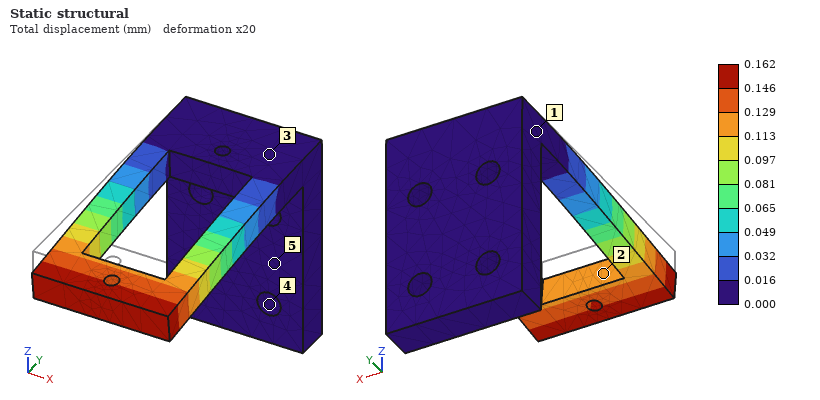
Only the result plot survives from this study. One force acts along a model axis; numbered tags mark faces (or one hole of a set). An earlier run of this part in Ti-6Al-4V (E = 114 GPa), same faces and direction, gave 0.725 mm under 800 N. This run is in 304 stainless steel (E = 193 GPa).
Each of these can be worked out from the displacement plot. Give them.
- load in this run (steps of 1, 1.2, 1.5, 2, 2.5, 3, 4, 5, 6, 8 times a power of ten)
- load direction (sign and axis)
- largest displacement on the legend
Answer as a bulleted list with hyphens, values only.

- 300 N
- -Z
- 0.162 mm
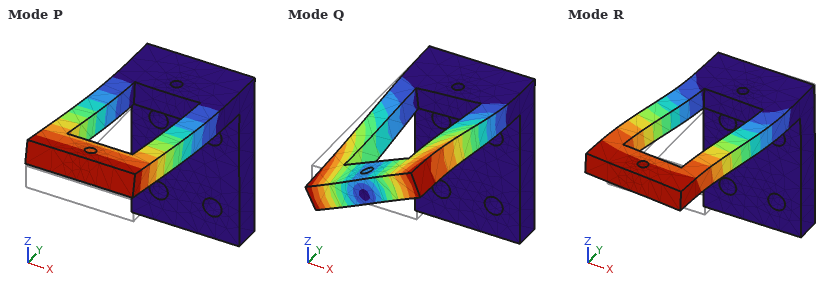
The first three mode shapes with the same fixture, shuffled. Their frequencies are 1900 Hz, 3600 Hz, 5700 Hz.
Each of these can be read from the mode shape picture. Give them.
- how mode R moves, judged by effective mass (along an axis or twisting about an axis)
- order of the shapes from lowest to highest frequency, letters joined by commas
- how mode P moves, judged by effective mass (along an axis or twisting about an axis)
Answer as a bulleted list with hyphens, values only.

- along X
- P, R, Q
- along Z
